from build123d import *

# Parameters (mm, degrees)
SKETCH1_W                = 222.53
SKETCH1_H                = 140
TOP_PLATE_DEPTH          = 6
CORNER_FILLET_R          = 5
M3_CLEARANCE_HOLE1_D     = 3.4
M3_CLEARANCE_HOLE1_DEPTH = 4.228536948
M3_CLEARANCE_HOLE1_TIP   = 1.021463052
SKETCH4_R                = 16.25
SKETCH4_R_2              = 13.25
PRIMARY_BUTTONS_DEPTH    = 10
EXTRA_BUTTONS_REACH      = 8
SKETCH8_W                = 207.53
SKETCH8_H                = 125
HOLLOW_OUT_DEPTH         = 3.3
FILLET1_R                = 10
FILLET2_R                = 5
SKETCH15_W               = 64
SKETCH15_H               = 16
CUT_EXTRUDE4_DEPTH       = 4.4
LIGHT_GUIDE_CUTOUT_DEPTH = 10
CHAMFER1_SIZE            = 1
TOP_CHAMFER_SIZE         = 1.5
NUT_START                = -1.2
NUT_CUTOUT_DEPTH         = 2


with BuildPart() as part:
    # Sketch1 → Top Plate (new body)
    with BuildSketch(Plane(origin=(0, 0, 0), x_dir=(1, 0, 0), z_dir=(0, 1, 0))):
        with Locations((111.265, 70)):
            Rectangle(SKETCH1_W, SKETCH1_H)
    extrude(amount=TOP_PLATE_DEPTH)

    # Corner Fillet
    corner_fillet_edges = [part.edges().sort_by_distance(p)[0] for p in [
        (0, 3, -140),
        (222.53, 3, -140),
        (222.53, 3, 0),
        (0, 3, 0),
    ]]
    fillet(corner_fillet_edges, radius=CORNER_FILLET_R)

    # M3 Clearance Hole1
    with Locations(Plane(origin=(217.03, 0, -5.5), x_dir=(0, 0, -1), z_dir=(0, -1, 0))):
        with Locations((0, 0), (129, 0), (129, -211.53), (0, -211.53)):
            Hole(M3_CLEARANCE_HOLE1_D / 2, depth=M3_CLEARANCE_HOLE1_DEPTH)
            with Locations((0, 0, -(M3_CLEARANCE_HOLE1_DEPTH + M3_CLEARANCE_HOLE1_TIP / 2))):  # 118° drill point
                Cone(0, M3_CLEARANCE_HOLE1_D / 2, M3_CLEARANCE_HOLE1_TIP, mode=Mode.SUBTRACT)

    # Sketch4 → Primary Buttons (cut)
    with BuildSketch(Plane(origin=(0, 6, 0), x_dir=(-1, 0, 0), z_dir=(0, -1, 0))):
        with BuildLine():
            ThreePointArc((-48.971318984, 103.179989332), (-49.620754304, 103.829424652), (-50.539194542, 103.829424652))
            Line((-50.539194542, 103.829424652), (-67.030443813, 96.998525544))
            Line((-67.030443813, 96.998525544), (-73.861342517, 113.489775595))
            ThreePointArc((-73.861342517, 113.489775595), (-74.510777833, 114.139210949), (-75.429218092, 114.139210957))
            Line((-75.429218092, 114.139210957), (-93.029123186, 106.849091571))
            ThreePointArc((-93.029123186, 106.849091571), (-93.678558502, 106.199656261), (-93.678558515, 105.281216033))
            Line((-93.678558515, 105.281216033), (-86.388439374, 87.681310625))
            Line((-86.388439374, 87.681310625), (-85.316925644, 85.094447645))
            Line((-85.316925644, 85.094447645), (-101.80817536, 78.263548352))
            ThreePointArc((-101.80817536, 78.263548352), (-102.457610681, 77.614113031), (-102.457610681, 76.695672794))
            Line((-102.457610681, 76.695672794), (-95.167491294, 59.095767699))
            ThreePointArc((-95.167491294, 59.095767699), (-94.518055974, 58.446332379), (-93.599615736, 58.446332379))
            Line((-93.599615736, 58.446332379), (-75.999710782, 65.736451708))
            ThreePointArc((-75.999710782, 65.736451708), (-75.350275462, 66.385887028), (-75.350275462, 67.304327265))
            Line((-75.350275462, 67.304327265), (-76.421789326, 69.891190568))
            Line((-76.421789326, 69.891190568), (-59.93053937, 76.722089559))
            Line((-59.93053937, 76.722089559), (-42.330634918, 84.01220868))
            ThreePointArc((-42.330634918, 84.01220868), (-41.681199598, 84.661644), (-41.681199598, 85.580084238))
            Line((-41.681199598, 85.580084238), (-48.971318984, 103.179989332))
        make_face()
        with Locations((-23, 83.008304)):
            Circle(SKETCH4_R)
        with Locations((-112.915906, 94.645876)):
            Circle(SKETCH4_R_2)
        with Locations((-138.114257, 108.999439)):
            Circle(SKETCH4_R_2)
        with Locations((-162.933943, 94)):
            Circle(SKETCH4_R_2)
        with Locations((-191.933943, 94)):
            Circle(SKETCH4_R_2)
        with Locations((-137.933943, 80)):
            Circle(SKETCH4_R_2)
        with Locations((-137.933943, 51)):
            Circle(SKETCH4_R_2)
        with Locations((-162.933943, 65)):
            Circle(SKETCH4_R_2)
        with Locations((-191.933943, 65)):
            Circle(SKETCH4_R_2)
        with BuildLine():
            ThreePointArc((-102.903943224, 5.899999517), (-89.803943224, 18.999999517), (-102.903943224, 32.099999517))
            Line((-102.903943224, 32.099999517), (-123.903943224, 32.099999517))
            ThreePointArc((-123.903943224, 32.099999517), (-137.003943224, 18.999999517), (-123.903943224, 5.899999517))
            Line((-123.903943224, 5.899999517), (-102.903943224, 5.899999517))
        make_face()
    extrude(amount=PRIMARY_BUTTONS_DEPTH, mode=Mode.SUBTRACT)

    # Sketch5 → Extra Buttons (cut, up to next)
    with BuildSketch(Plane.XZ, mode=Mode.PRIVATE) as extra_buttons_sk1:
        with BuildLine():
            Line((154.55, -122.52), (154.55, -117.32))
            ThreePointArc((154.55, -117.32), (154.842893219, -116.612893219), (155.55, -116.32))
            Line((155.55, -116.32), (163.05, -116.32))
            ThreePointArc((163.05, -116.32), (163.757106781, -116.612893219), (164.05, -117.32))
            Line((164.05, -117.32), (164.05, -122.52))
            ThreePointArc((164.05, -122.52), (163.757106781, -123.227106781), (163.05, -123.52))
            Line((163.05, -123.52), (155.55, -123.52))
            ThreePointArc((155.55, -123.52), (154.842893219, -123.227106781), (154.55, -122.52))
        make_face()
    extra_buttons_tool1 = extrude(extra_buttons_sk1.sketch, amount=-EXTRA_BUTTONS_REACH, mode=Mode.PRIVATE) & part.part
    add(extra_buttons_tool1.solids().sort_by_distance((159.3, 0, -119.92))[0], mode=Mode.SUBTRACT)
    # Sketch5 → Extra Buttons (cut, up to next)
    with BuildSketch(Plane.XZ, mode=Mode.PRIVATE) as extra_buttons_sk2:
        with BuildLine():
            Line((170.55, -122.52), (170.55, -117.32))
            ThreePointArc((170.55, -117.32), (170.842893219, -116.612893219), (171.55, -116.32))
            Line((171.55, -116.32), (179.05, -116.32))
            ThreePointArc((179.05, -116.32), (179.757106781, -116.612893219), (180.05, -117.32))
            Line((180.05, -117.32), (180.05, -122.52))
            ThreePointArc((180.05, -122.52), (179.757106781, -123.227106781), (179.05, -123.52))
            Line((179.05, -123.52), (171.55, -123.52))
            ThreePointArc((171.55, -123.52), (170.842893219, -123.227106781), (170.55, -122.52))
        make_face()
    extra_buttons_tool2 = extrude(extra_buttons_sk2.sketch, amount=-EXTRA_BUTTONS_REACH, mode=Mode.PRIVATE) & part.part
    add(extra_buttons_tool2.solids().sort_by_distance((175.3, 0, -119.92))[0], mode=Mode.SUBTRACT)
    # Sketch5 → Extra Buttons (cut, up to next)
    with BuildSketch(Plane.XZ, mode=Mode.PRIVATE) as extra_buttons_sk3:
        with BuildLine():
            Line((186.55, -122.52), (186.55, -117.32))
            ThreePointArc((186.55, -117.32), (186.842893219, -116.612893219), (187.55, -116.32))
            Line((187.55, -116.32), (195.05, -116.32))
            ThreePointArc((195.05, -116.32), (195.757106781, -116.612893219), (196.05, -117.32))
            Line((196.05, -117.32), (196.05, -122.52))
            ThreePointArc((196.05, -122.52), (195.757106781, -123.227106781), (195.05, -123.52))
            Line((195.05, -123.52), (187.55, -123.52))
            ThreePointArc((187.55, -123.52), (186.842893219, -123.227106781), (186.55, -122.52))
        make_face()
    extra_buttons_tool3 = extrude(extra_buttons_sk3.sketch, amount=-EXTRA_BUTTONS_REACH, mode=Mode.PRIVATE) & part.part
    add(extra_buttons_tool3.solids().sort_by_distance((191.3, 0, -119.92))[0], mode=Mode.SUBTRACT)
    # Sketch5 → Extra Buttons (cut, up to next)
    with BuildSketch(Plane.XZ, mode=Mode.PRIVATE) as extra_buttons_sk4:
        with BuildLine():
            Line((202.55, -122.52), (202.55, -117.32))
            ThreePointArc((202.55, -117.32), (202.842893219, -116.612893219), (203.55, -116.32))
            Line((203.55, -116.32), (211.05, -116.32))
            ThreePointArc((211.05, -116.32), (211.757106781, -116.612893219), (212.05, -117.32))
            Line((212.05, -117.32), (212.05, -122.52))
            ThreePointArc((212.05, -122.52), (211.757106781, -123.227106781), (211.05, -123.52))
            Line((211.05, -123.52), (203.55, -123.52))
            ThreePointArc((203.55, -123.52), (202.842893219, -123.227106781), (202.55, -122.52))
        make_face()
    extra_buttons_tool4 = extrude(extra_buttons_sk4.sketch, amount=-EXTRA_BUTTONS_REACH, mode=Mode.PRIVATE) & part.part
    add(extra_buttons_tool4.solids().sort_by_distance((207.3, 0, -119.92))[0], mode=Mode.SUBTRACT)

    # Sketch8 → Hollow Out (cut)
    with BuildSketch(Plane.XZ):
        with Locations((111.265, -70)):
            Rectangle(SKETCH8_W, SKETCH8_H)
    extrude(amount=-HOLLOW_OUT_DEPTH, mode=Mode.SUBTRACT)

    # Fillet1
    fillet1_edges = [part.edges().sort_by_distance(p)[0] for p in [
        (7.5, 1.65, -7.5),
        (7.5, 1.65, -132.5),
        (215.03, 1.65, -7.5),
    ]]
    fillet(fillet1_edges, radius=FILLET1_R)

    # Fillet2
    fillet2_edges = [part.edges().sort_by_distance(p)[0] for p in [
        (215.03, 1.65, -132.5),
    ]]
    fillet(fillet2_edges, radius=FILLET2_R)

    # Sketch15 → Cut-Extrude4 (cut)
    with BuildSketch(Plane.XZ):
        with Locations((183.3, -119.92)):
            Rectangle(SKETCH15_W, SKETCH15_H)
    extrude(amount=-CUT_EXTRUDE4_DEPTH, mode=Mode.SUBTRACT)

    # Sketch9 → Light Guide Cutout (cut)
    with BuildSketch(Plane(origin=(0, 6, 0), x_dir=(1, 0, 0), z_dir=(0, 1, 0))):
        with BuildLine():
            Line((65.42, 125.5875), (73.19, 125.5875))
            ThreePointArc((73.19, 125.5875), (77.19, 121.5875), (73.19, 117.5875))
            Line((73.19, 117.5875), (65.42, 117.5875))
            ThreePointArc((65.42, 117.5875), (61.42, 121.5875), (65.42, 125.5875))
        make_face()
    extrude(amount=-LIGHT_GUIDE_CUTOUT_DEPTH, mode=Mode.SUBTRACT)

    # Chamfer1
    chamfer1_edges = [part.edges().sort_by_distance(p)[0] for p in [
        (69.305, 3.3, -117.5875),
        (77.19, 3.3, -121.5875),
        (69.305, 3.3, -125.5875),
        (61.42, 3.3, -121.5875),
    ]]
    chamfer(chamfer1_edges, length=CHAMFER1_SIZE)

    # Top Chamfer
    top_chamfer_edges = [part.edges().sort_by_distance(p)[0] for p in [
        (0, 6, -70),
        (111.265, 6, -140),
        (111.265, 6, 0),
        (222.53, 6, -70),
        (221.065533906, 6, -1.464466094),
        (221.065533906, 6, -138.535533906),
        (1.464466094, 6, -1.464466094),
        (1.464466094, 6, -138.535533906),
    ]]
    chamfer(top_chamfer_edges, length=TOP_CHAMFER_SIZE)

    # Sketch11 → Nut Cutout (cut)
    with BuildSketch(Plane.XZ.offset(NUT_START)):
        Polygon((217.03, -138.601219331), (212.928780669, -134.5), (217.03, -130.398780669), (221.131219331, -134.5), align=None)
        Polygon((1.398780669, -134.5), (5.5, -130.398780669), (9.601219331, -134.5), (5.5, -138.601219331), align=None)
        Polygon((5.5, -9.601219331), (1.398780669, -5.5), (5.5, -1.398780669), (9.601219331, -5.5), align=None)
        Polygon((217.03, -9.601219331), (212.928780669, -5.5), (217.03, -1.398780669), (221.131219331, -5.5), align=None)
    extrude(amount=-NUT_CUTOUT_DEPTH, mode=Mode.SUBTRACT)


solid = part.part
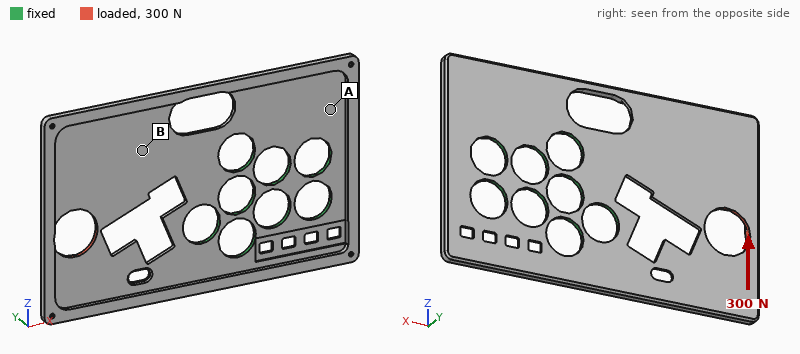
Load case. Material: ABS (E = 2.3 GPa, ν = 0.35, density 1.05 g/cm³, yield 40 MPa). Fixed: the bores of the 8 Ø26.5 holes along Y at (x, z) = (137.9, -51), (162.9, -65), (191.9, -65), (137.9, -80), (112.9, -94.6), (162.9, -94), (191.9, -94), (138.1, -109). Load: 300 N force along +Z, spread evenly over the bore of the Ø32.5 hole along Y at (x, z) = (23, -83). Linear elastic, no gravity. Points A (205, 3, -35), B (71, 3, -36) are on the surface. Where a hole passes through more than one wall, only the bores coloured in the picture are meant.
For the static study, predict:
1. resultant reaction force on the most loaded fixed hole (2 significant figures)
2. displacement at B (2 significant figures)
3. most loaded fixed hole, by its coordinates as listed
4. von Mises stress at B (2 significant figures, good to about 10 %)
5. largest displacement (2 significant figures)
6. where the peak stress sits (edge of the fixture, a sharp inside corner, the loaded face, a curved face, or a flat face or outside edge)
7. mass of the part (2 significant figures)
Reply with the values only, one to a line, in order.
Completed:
350 N
0.60 mm
(112.9, -94.6)
3.0 MPa
2.7 mm
a curved face
80 g
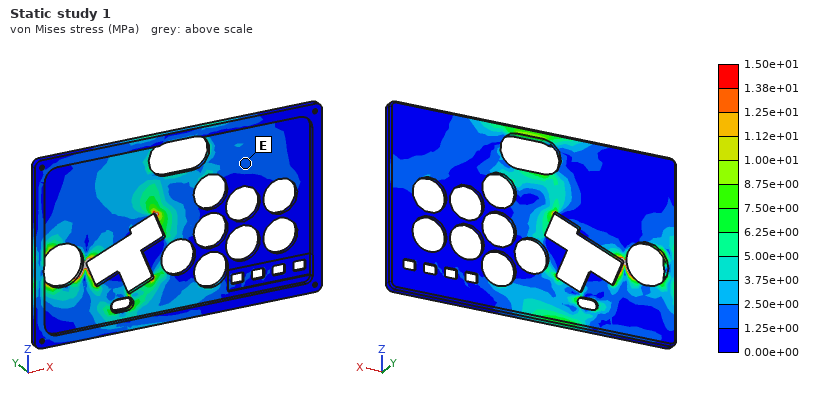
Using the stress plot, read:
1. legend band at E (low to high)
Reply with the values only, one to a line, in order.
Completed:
1.25e+00 to 2.50e+00 MPa
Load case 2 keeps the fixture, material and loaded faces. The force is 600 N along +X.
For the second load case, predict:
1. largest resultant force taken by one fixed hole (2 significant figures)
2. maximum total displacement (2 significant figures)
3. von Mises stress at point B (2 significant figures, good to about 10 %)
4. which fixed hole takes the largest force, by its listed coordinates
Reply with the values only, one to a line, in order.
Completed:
320 N
0.77 mm
1.7 MPa
(137.9, -51)
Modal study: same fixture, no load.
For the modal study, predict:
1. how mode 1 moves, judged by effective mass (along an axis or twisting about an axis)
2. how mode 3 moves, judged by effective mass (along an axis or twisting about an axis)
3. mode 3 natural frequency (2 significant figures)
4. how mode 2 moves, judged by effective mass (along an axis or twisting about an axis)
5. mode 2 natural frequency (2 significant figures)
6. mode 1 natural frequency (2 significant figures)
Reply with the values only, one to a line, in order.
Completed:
along Y
along Y
250 Hz
twisting about X
93 Hz
47 Hz
